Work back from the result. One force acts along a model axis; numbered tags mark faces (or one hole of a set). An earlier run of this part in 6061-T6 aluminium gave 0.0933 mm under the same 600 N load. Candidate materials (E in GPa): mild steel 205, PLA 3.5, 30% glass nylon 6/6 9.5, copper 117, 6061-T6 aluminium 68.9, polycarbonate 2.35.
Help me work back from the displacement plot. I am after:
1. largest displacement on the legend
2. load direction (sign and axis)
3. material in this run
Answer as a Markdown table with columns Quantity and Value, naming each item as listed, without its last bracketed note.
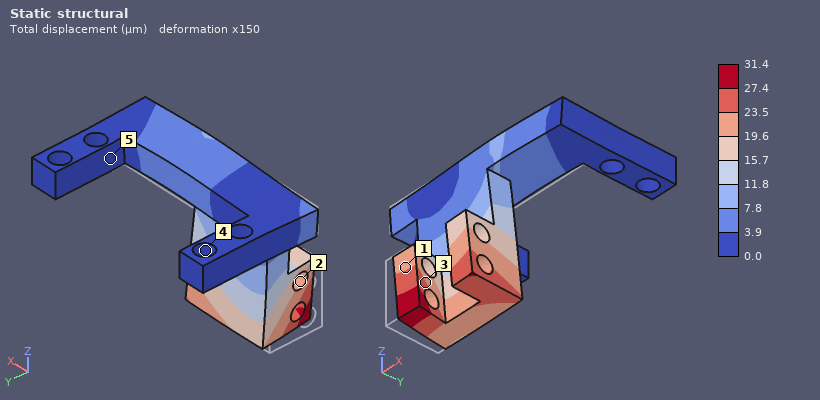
| Quantity | Value |
|---|---|
| largest displacement on the legend | 31.4 µm |
| load direction | +X |
| material in this run | mild steel |
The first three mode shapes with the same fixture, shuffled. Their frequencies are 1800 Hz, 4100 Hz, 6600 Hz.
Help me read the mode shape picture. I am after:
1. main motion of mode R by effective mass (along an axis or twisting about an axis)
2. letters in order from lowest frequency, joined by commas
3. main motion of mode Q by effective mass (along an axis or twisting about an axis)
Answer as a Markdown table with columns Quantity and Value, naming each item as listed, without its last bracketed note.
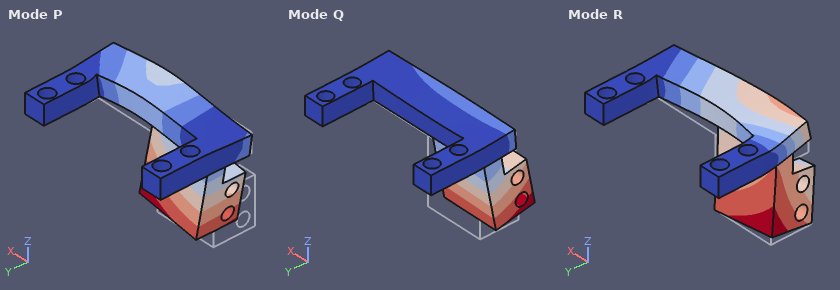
| Quantity | Value |
|---|---|
| main motion of mode R by effective mass | along Z |
| letters in order from lowest frequency, joined by commas | Q, P, R |
| main motion of mode Q by effective mass | along Y |
